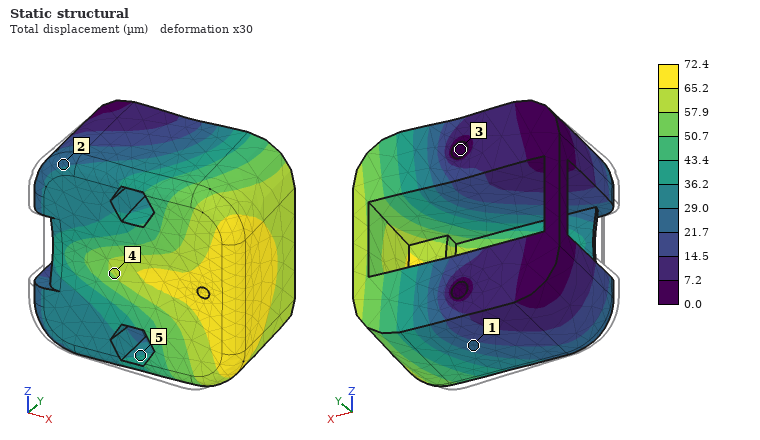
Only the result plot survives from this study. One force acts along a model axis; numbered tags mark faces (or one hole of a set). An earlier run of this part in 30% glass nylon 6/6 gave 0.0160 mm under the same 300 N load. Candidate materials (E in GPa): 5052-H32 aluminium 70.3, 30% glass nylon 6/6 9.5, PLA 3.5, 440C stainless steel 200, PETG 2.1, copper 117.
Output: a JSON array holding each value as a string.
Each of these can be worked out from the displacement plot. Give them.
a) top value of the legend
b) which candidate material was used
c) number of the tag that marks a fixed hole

["72.4 µm", "PETG", "3"]
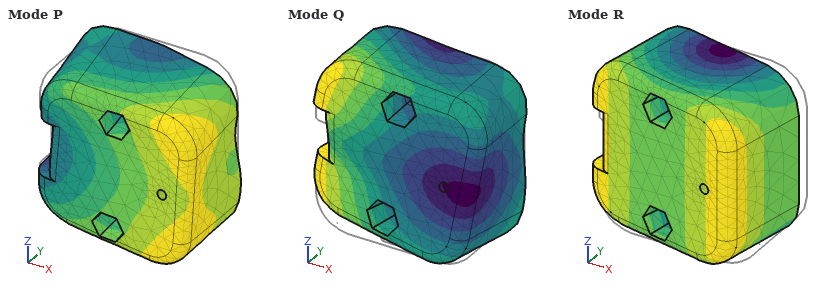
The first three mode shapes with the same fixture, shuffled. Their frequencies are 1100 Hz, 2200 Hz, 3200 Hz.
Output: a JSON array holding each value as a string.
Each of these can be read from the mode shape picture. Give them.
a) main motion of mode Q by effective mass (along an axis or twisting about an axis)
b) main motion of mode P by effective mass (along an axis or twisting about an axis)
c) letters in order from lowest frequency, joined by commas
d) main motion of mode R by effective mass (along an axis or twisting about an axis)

["along Z", "along Z", "R, Q, P", "along X"]
